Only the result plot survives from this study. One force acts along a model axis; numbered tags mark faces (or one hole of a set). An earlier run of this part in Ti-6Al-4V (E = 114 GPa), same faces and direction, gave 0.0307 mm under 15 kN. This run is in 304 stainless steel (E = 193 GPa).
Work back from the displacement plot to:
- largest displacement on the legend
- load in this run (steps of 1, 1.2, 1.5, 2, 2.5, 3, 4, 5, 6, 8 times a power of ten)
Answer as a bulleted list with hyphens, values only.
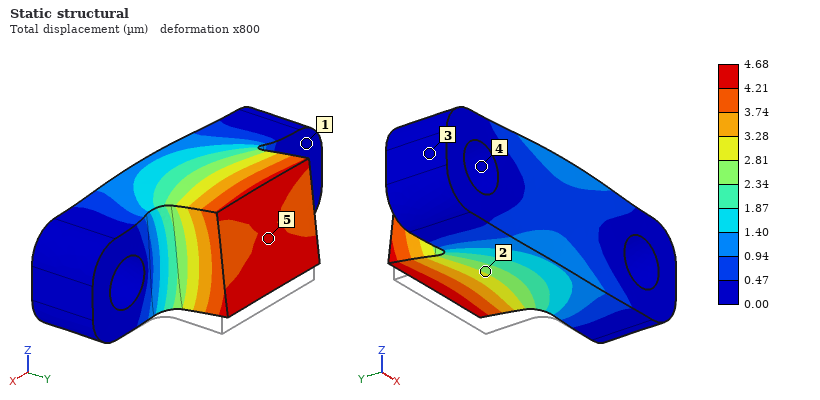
- 4.68 µm
- 4 kN
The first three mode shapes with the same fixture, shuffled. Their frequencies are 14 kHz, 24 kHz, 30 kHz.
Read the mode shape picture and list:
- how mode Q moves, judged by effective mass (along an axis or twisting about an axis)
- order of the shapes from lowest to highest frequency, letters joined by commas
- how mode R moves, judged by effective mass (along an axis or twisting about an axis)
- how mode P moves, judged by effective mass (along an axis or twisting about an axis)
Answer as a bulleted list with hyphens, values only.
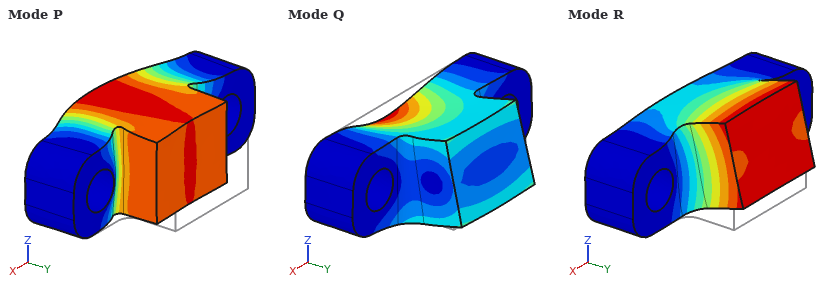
- along Z
- R, P, Q
- along Z
- along Y
